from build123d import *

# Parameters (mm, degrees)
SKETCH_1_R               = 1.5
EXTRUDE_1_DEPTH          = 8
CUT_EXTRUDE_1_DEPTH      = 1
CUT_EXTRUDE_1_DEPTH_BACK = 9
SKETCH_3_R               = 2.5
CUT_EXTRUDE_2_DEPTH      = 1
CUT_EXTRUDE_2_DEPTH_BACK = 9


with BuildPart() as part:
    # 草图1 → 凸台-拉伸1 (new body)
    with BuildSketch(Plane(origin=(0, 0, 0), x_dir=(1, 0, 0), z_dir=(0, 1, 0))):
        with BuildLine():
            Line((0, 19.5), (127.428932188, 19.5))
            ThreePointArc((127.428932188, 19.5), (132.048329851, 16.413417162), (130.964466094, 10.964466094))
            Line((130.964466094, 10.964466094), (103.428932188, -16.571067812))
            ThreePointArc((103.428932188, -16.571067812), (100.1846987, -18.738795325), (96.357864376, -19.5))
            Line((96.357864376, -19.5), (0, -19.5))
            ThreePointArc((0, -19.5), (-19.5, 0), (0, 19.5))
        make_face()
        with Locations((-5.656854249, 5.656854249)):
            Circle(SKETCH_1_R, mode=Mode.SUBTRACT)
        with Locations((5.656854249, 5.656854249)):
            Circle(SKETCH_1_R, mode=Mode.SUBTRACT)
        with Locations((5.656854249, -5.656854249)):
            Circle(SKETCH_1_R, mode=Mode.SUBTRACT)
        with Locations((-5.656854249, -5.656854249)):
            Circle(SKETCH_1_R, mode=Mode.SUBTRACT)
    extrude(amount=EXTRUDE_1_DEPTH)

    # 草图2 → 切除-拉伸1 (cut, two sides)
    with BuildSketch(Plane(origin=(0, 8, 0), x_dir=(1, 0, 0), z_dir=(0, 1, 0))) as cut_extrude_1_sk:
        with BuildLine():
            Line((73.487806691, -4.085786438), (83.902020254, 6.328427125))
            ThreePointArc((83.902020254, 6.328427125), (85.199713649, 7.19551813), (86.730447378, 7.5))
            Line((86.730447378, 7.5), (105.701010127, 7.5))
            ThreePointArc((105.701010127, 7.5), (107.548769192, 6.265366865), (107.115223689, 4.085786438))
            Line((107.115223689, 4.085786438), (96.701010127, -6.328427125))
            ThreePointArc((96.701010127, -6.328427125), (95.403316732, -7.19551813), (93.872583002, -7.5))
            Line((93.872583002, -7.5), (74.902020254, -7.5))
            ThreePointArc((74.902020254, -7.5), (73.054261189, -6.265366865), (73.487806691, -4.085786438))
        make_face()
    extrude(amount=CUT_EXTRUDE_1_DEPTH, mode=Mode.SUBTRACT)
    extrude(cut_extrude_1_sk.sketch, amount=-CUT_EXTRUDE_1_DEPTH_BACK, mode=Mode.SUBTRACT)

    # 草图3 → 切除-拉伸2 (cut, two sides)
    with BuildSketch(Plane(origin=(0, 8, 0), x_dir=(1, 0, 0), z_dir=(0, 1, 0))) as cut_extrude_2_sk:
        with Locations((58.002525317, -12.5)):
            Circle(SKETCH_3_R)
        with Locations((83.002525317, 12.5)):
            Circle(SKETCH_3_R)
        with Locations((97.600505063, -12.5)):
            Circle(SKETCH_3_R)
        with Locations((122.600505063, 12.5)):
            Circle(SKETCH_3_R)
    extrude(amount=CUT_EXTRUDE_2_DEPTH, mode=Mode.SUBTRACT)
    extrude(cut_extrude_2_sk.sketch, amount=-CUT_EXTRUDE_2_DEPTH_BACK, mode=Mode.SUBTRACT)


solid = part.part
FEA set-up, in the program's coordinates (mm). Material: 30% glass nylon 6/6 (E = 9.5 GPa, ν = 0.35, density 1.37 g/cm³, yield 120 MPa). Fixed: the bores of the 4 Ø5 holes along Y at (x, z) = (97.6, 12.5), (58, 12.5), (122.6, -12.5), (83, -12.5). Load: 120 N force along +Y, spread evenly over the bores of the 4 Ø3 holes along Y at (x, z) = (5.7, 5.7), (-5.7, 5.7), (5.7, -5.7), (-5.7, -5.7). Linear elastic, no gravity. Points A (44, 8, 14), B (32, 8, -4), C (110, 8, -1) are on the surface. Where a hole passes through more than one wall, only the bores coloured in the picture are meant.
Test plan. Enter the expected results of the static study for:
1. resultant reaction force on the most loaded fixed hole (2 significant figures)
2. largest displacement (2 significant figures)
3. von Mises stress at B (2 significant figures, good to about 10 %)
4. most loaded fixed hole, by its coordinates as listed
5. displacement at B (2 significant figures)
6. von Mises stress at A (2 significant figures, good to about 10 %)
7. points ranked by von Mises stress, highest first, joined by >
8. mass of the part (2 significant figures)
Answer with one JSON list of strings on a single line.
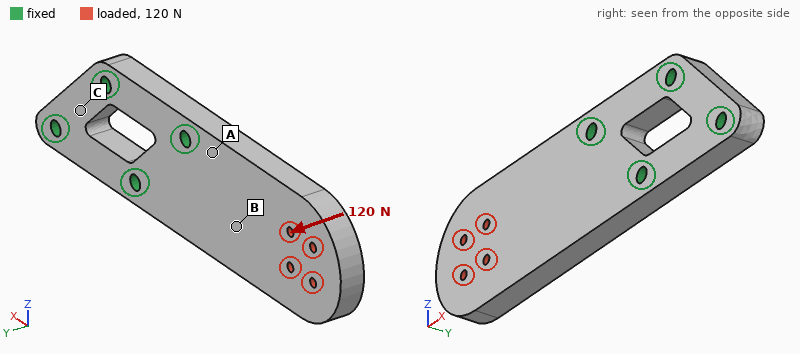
["210 N", "0.89 mm", "8.7 MPa", "(58, 12.5)", "0.20 mm", "15 MPa", "A > B > C", "52 g"]
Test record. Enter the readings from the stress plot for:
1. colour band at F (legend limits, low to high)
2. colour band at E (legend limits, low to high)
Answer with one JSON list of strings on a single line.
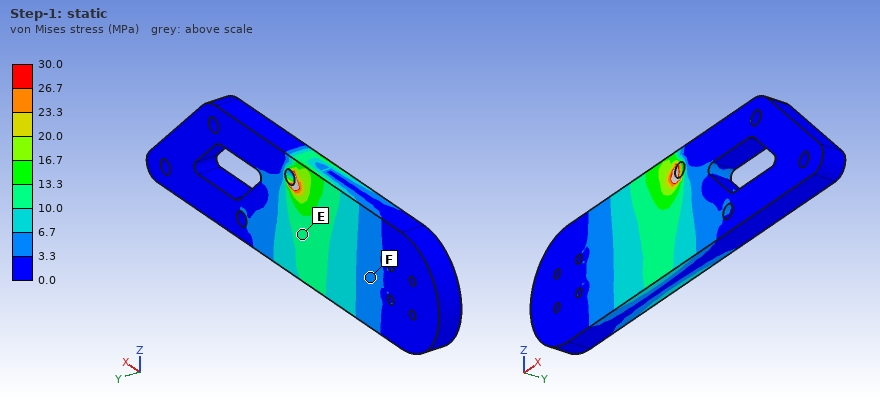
["3.3 to 6.7 MPa", "10.0 to 13.3 MPa"]
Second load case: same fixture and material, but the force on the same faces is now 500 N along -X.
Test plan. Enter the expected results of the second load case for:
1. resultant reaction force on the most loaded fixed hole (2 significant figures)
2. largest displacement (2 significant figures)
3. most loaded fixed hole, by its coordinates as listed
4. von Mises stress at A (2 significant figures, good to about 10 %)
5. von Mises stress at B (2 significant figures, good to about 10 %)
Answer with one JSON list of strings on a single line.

["260 N", "20 µm", "(58, 12.5)", "1.7 MPa", "1.6 MPa"]
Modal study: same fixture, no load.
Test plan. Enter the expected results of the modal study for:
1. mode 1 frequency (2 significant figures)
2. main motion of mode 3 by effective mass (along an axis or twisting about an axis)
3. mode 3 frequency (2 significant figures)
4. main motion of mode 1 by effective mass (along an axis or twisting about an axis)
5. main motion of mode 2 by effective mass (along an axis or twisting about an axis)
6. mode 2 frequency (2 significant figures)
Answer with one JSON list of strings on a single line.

["570 Hz", "along Z", "2100 Hz", "along Y", "twisting about X", "2000 Hz"]
